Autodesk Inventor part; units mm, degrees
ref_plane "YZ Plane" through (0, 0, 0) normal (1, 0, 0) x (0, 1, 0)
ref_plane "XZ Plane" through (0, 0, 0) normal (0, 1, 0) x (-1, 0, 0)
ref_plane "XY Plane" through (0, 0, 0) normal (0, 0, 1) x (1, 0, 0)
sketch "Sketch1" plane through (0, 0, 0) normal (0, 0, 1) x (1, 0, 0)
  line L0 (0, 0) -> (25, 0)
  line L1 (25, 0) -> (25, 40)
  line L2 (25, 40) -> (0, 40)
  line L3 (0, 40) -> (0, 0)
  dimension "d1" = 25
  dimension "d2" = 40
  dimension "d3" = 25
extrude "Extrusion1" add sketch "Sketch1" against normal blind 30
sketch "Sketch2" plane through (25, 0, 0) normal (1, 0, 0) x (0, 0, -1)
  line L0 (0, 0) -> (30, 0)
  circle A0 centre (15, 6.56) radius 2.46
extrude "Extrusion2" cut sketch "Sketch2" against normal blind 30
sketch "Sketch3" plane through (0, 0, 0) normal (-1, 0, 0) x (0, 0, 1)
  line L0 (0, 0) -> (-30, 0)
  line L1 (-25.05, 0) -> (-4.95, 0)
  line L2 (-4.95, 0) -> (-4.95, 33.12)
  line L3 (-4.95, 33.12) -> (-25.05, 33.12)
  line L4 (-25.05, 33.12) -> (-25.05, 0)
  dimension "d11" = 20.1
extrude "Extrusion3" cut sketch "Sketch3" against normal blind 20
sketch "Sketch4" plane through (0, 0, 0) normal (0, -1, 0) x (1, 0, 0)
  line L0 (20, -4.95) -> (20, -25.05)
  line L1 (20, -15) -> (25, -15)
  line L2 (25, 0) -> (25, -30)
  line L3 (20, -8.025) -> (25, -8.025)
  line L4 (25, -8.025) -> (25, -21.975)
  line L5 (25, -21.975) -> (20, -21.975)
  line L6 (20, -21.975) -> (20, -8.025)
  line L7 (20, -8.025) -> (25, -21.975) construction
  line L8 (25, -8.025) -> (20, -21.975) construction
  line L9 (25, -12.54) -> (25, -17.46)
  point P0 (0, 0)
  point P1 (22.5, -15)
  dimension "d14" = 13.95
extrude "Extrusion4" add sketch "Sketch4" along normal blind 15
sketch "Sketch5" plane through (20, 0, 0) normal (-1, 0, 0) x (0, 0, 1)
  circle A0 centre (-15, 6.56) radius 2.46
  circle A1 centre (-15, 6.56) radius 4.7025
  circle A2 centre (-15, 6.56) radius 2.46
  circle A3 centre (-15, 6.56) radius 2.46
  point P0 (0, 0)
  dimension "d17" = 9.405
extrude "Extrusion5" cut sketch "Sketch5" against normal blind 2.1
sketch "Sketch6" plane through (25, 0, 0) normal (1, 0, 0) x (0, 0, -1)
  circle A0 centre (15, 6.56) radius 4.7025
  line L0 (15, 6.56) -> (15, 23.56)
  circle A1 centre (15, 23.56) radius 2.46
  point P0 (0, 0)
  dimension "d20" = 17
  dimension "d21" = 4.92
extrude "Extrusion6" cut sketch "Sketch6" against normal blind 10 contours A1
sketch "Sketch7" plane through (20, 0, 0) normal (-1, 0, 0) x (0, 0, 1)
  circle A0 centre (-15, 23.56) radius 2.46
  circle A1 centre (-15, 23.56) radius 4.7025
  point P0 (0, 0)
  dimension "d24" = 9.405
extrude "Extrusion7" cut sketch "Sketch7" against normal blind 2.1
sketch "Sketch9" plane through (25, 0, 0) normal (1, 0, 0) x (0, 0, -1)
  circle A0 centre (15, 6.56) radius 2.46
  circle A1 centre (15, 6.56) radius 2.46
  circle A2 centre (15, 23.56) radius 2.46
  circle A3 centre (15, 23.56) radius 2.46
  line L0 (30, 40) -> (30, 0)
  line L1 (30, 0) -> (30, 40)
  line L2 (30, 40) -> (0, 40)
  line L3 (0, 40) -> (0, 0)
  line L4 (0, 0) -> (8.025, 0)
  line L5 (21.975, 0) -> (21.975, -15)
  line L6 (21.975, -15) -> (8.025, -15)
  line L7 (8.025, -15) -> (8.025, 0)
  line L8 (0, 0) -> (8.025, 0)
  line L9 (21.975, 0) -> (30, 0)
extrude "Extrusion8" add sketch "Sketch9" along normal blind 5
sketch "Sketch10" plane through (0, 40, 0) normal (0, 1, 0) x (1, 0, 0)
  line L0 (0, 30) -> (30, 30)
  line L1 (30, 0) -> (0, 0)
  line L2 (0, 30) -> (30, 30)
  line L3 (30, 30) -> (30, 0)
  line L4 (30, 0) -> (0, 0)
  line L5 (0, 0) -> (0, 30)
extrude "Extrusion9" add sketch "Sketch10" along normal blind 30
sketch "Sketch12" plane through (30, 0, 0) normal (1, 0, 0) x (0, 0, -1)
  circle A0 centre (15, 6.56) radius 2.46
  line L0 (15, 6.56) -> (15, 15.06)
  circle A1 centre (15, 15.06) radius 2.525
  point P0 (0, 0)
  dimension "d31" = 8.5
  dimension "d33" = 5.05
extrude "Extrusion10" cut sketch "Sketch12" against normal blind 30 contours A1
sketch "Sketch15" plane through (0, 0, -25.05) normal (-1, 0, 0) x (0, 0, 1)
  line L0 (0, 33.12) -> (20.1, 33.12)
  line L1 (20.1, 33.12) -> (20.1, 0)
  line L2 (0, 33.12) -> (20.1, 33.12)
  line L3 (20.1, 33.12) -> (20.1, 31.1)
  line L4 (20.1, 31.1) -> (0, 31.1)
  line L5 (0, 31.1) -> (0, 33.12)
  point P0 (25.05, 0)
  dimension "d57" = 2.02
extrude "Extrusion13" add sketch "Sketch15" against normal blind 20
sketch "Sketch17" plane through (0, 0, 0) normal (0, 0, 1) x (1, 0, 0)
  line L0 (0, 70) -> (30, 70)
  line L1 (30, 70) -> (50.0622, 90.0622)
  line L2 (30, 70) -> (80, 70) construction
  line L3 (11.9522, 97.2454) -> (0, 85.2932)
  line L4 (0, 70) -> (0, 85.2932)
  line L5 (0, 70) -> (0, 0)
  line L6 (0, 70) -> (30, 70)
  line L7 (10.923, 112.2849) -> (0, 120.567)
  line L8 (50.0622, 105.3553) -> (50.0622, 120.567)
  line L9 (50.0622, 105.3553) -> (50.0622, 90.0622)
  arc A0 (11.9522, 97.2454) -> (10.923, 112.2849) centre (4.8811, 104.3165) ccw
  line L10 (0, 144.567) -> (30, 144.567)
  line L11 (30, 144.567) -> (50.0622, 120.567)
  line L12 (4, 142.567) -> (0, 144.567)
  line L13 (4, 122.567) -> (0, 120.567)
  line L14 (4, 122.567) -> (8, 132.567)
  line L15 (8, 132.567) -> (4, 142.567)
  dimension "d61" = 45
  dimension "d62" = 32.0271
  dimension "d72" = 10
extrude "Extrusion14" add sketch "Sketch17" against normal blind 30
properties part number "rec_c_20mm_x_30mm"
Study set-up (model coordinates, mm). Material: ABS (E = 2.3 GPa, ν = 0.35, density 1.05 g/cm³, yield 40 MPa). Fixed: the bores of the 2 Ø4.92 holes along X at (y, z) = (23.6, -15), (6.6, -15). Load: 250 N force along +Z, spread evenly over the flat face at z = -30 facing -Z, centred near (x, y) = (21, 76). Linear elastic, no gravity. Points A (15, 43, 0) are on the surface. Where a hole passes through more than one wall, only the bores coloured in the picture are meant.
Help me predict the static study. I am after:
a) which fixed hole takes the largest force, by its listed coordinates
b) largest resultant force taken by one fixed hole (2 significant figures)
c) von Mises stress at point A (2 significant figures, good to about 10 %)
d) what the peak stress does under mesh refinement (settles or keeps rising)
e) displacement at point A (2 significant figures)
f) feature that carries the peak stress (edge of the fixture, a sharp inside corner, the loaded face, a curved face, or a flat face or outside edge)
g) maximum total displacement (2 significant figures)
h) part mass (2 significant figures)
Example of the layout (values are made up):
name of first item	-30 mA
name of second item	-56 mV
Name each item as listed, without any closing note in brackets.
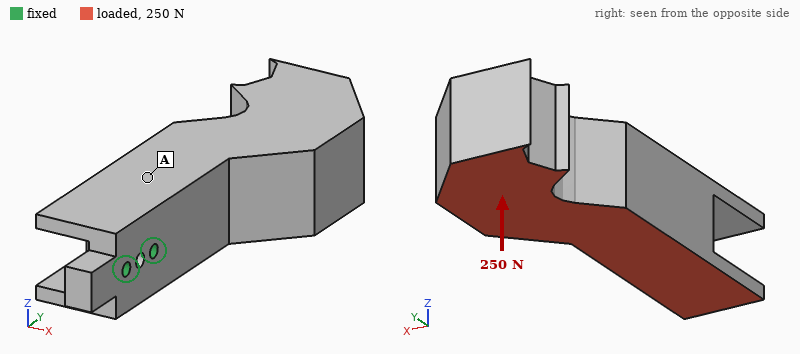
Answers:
which fixed hole takes the largest force, by its listed coordinates	(23.6, -15)
largest resultant force taken by one fixed hole	810 N
von Mises stress at point A	2.3 MPa
what the peak stress does under mesh refinement	keeps rising
displacement at point A	0.17 mm
feature that carries the peak stress	edge of the fixture
maximum total displacement	1.0 mm
part mass	140 g
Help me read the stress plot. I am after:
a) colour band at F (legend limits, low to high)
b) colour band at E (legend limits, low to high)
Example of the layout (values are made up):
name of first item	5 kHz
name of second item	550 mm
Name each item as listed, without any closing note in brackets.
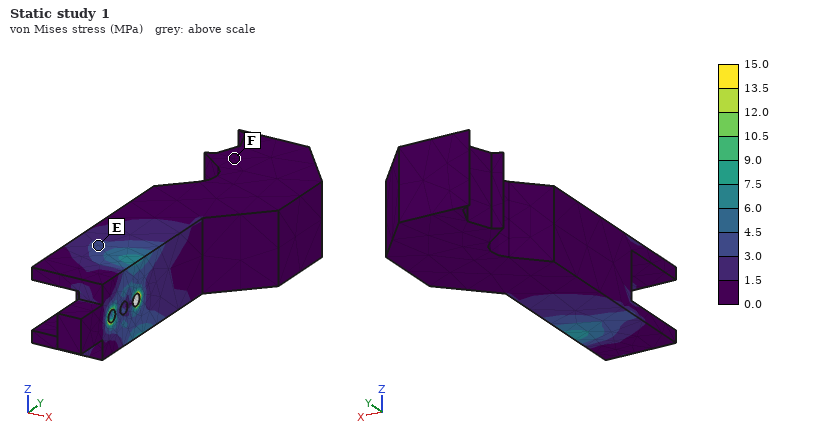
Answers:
colour band at F	0.0 to 1.5 MPa
colour band at E	3.0 to 4.5 MPa
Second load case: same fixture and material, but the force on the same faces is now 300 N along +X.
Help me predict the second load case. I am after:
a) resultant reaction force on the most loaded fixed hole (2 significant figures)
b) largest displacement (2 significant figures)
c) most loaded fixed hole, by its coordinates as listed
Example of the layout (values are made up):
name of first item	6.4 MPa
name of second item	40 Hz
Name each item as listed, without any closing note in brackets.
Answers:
resultant reaction force on the most loaded fixed hole	900 N
largest displacement	1.8 mm
most loaded fixed hole, by its coordinates as listed	(23.6, -15)
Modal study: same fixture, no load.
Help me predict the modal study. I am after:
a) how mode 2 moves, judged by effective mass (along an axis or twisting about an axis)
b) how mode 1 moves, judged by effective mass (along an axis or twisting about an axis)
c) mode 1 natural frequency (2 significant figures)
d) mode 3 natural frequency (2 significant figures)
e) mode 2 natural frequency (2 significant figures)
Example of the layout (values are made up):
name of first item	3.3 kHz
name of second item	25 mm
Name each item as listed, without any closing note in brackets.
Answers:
how mode 2 moves, judged by effective mass	along Z
how mode 1 moves, judged by effective mass	along X
mode 1 natural frequency	210 Hz
mode 3 natural frequency	680 Hz
mode 2 natural frequency	240 Hz
